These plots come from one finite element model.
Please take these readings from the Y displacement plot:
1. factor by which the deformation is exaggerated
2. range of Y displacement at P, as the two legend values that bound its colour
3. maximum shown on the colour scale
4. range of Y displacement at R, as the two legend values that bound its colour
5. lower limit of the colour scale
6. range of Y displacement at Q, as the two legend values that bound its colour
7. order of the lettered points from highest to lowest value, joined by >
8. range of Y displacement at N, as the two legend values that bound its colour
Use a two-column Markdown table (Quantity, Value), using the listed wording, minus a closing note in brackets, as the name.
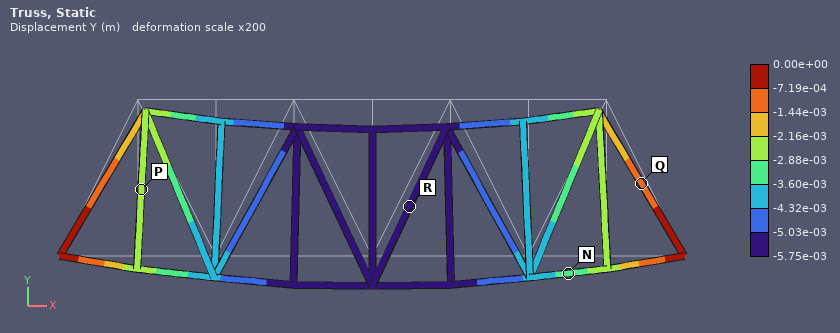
| Quantity | Value |
|---|---|
| factor by which the deformation is exaggerated | 200 |
| range of Y displacement at P, as the two legend values that bound its colour | -2.88e-03 to -2.16e-03 m |
| maximum shown on the colour scale | 0.00e+00 m |
| range of Y displacement at R, as the two legend values that bound its colour | -5.75e-03 to -5.03e-03 m |
| lower limit of the colour scale | -5.75e-03 m |
| range of Y displacement at Q, as the two legend values that bound its colour | -1.44e-03 to -7.19e-04 m |
| order of the lettered points from highest to lowest value, joined by > | Q > P > N > R |
| range of Y displacement at N, as the two legend values that bound its colour | -3.60e-03 to -2.88e-03 m |
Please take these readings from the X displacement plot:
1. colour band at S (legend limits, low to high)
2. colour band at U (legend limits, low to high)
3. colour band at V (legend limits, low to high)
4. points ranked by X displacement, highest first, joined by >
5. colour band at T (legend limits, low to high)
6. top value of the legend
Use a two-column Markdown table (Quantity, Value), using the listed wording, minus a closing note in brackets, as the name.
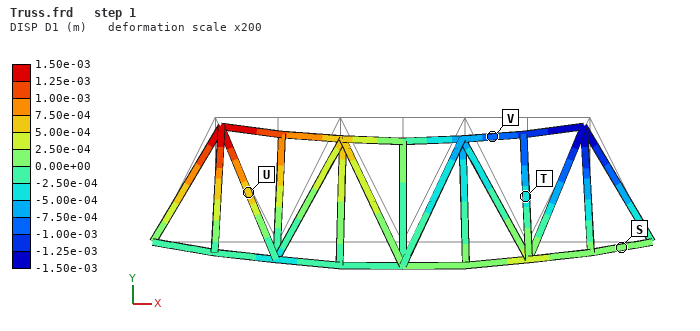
| Quantity | Value |
|---|---|
| colour band at S | 0.00e+00 to 2.50e-04 m |
| colour band at U | 5.00e-04 to 7.50e-04 m |
| colour band at V | -1.00e-03 to -7.50e-04 m |
| points ranked by X displacement, highest first, joined by > | U > S > T > V |
| colour band at T | -5.00e-04 to -2.50e-04 m |
| top value of the legend | 1.50e-03 m |
